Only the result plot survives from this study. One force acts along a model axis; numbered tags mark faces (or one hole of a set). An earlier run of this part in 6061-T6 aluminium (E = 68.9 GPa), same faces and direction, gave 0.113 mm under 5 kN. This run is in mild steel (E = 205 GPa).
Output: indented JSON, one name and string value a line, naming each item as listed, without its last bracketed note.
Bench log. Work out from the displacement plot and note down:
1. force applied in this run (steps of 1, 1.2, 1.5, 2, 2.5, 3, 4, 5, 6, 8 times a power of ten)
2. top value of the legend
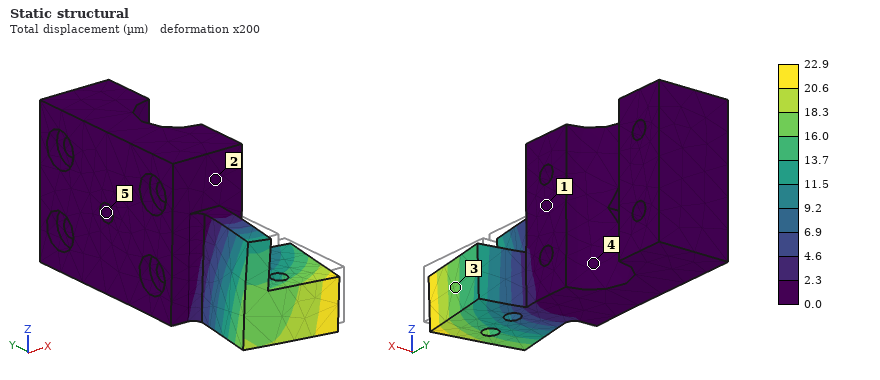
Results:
{
  "force applied in this run": "3 kN",
  "top value of the legend": "22.9 µm"
}
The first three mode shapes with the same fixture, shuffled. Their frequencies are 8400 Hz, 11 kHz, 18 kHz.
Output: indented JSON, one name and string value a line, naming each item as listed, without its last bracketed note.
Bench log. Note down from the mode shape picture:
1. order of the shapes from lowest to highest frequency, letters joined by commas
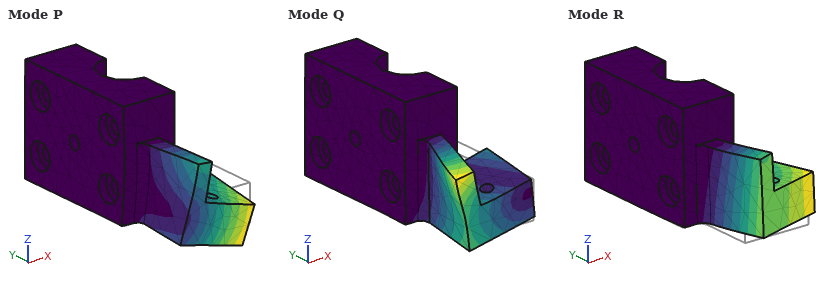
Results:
{
  "order of the shapes from lowest to highest frequency, letters joined by commas": "R, P, Q"
}
